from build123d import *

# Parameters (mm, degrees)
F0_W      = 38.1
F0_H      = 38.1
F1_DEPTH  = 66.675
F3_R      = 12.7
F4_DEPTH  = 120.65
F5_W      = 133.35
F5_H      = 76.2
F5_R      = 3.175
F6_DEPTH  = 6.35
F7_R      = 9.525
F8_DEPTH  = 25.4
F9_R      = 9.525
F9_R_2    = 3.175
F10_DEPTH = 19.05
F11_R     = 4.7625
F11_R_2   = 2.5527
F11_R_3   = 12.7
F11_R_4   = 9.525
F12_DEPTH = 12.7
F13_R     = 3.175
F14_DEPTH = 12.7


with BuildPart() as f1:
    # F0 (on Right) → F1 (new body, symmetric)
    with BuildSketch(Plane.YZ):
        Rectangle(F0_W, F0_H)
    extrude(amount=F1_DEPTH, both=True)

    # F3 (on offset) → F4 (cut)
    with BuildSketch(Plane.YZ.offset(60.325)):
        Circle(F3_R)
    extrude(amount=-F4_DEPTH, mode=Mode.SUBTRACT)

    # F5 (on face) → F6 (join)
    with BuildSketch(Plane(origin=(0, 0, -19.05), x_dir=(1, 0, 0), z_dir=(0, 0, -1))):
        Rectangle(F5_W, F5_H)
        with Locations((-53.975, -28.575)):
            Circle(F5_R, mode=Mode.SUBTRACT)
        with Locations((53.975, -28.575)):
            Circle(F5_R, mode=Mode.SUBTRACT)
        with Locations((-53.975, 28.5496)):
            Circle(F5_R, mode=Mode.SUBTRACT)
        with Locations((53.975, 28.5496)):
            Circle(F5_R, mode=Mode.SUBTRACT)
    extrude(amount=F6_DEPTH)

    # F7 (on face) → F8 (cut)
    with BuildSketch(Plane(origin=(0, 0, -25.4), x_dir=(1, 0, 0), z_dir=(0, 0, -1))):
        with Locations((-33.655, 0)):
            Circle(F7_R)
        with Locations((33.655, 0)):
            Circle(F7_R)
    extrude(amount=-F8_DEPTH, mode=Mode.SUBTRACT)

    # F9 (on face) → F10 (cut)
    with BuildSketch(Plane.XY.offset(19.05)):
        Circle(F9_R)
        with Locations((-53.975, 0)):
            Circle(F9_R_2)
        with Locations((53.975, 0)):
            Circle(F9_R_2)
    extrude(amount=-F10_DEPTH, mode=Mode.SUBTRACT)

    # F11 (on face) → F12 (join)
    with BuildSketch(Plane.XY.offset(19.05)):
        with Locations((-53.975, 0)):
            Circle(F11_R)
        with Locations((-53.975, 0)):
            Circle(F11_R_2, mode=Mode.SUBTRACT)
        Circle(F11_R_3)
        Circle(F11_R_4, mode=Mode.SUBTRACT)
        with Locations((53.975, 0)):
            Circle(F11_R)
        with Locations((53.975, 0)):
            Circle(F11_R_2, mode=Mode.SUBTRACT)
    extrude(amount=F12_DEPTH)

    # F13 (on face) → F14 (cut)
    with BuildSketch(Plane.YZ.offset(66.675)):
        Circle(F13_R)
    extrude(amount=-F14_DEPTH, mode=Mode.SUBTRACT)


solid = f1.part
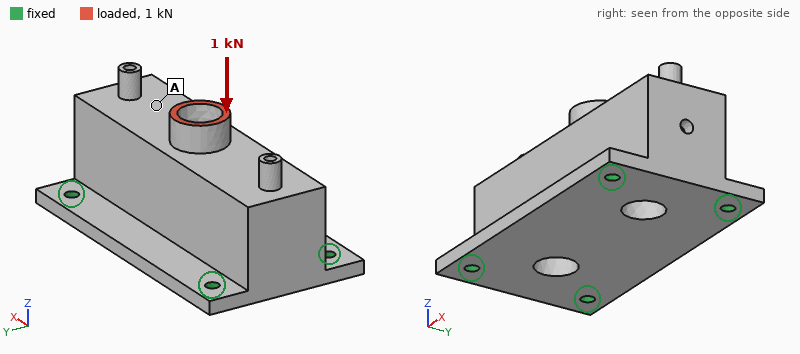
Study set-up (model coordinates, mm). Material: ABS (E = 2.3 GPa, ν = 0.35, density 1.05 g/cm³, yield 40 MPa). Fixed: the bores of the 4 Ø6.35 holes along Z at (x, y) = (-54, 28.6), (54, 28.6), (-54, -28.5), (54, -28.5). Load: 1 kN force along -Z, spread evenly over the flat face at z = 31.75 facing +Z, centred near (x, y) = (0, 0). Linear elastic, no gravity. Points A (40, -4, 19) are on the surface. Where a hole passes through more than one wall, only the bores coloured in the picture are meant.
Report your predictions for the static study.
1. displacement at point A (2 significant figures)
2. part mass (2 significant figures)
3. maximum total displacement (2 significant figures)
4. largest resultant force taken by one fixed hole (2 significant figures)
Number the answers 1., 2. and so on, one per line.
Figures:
1. 0.082 mm
2. 200 g
3. 0.18 mm
4. 300 N
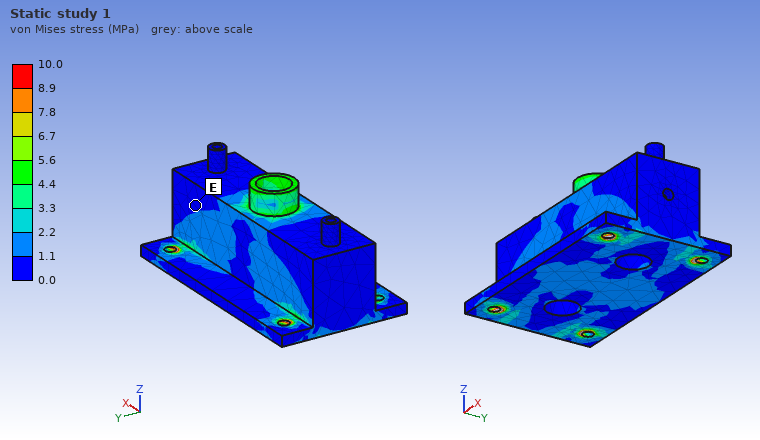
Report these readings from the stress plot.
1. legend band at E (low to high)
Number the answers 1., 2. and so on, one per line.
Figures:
1. 0.0 to 1.1 MPa
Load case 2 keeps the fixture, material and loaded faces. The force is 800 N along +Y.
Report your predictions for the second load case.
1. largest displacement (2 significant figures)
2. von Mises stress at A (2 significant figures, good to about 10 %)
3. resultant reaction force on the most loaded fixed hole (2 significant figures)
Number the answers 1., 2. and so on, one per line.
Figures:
1. 0.65 mm
2. 2.5 MPa
3. 510 N
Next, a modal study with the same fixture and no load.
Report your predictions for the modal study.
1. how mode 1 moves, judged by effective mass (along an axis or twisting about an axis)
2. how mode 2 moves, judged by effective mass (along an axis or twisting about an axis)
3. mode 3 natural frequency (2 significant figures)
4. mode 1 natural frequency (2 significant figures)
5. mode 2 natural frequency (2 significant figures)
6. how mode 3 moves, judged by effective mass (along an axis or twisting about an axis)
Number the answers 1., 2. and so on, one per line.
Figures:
1. along Y
2. along Z
3. 1700 Hz
4. 1200 Hz
5. 1300 Hz
6. along X
